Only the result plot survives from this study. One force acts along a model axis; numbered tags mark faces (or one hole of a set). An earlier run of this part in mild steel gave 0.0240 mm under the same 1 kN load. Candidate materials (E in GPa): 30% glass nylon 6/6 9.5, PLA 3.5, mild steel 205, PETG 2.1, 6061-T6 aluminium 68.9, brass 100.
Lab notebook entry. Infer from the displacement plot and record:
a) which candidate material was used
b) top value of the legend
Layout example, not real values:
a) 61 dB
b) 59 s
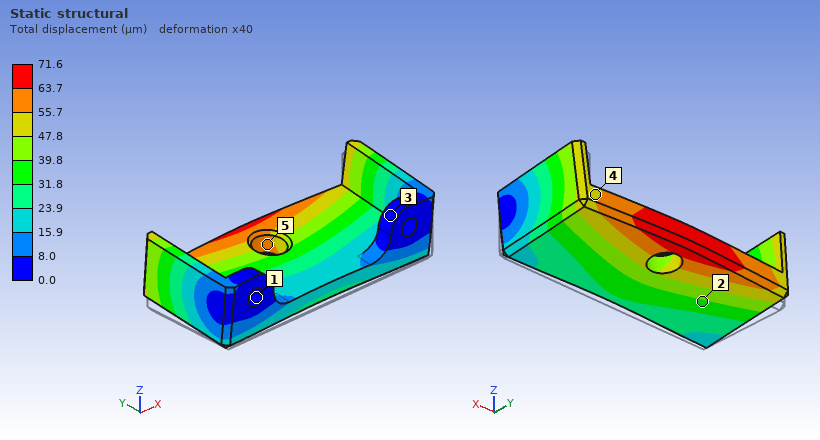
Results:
a) 6061-T6 aluminium
b) 71.6 µm
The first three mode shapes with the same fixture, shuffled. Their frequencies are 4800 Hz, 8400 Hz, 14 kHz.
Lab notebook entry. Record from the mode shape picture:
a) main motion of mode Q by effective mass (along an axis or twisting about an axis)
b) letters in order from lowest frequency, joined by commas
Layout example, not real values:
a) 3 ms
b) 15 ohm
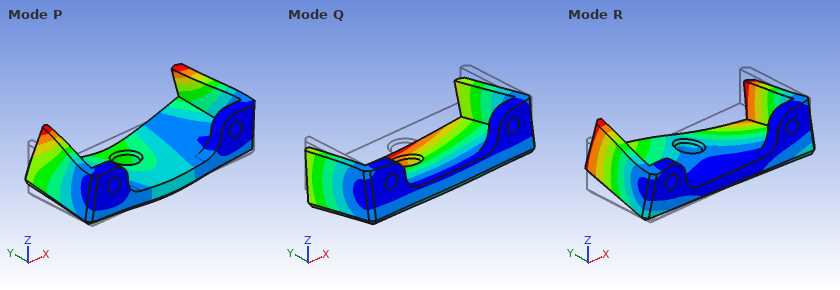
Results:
a) along Z
b) Q, R, P
